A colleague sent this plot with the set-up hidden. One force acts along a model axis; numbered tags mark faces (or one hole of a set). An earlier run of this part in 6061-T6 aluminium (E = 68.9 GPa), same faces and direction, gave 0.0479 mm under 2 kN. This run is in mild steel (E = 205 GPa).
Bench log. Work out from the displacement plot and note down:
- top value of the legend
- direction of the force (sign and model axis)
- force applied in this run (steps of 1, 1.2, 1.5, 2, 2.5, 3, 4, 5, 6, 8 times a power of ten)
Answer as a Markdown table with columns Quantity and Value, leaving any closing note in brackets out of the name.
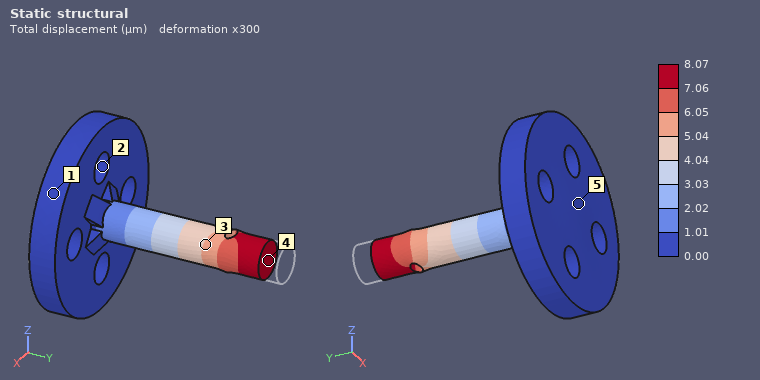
| Quantity | Value |
|---|---|
| top value of the legend | 8.07 µm |
| direction of the force | -Y |
| force applied in this run | 1 kN |
